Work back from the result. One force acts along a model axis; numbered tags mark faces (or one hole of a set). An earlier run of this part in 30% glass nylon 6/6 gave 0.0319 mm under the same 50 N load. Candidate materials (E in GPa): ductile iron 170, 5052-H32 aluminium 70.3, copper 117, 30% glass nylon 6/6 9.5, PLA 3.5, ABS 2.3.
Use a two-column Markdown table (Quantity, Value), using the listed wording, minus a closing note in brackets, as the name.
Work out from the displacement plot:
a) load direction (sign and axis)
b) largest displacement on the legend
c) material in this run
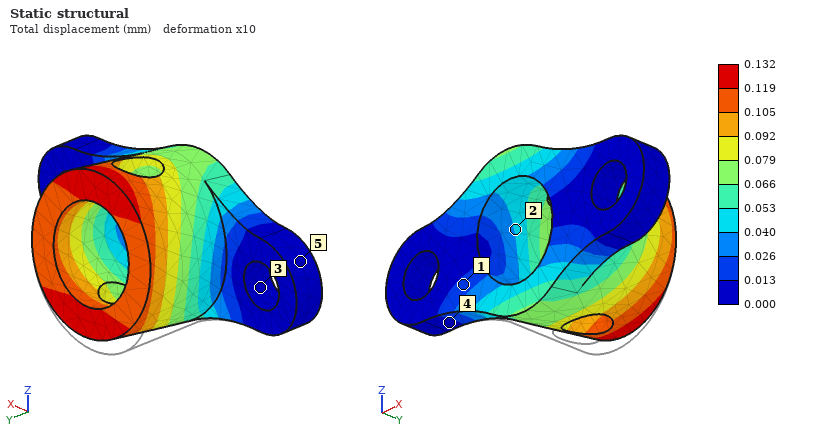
| Quantity | Value |
|---|---|
| load direction | +Z |
| largest displacement on the legend | 0.132 mm |
| material in this run | ABS |
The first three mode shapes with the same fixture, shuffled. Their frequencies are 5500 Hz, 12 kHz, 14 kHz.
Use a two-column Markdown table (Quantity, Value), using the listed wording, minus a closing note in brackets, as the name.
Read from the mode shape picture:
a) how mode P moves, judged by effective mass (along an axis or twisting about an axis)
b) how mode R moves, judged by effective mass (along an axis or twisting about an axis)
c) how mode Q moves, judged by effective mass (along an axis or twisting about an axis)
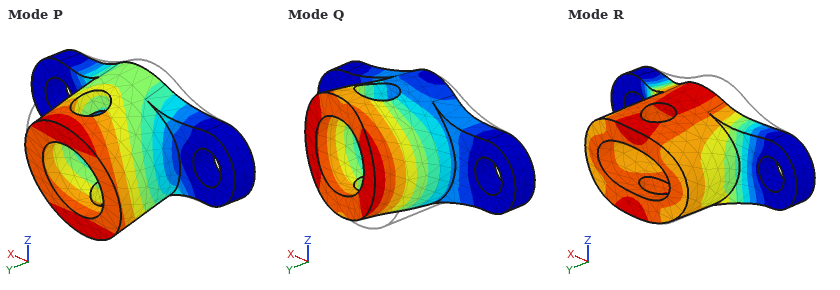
| Quantity | Value |
|---|---|
| how mode P moves, judged by effective mass | along Z |
| how mode R moves, judged by effective mass | along Y |
| how mode Q moves, judged by effective mass | along X |
